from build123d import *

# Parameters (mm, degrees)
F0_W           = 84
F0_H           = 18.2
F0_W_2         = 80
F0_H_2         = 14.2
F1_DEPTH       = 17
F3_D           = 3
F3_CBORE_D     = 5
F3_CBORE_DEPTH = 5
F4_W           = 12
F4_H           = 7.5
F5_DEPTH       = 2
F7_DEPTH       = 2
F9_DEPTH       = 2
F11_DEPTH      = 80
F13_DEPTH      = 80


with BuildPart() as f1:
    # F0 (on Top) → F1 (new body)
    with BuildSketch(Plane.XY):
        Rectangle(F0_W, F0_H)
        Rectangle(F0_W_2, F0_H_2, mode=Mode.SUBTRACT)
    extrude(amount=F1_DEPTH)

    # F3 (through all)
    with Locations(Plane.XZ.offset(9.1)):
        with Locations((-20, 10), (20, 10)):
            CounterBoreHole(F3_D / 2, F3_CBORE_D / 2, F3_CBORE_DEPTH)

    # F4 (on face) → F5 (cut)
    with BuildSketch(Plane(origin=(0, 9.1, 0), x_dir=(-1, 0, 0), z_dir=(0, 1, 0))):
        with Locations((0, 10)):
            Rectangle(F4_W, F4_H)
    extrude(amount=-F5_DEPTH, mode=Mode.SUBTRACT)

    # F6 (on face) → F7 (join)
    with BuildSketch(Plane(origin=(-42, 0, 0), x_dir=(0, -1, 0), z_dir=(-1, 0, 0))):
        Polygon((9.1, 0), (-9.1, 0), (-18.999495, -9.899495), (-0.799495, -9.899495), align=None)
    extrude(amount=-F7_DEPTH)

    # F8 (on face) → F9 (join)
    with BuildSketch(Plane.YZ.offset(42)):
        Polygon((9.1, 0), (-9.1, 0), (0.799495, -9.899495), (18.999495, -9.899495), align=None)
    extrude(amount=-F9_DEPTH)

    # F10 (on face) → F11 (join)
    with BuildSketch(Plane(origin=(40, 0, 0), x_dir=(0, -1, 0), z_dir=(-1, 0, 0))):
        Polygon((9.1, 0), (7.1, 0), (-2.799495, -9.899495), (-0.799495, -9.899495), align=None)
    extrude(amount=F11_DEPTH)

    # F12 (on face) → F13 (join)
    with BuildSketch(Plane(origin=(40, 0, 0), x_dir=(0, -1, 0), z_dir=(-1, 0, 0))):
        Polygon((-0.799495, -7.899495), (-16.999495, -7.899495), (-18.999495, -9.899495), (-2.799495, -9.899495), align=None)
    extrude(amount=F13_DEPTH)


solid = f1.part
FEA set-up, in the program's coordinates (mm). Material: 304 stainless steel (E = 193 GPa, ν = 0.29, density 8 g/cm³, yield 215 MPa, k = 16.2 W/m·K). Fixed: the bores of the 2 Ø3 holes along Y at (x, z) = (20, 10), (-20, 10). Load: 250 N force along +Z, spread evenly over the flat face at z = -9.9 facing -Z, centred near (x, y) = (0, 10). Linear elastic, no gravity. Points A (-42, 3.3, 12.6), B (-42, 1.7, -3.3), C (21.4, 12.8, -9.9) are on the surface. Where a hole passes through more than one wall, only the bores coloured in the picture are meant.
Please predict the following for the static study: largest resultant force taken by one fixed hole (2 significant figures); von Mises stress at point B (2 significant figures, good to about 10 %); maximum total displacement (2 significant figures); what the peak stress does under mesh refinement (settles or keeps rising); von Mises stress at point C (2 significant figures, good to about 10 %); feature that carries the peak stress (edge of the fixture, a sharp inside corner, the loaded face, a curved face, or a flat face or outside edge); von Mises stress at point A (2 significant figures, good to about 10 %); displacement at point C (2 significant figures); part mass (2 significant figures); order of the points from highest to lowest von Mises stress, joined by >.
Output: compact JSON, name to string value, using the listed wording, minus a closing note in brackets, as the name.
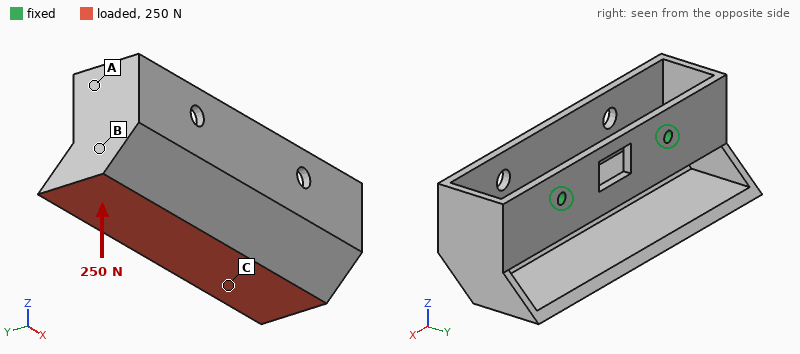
{"largest resultant force taken by one fixed hole": "150 N", "von Mises stress at point B": "20 MPa", "maximum total displacement": "0.12 mm", "what the peak stress does under mesh refinement": "keeps rising", "von Mises stress at point C": "32 MPa", "feature that carries the peak stress": "edge of the fixture", "von Mises stress at point A": "7.6 MPa", "displacement at point C": "0.065 mm", "part mass": "90 g", "order of the points from highest to lowest von Mises stress, joined by >": "C > B > A"}
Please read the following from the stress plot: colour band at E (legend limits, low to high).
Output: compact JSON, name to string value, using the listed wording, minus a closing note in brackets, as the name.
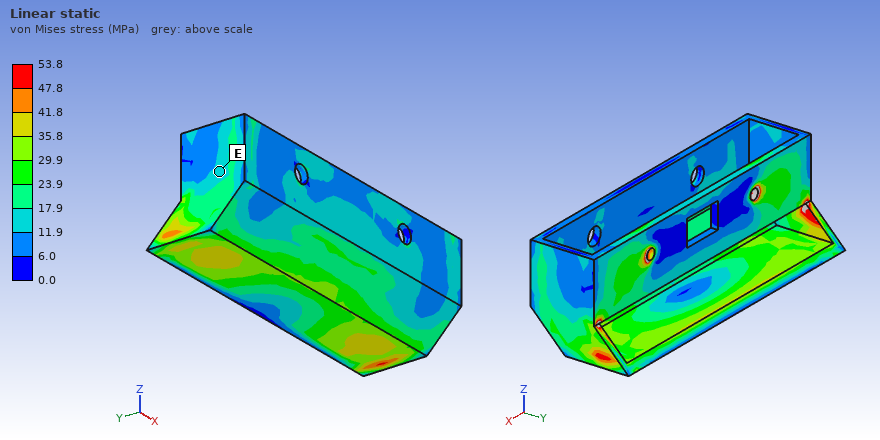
{"colour band at E": "11.9 to 17.9 MPa"}
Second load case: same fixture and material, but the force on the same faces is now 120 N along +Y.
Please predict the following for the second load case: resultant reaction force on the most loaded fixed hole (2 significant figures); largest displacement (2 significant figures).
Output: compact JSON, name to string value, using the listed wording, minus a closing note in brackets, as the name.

{"resultant reaction force on the most loaded fixed hole": "64 N", "largest displacement": "0.17 mm"}
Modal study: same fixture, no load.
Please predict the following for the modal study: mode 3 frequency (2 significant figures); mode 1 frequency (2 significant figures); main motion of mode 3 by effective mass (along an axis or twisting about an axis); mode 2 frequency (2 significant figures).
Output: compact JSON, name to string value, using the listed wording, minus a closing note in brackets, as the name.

{"mode 3 frequency": "1300 Hz", "mode 1 frequency": "640 Hz", "main motion of mode 3 by effective mass": "along Y", "mode 2 frequency": "940 Hz"}
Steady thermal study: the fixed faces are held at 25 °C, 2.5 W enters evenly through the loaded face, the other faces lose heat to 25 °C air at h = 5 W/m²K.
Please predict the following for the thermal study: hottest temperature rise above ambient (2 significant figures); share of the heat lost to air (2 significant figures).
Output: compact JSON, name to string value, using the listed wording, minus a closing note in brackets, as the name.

{"hottest temperature rise above ambient": "49 K", "share of the heat lost to air": "61 %"}
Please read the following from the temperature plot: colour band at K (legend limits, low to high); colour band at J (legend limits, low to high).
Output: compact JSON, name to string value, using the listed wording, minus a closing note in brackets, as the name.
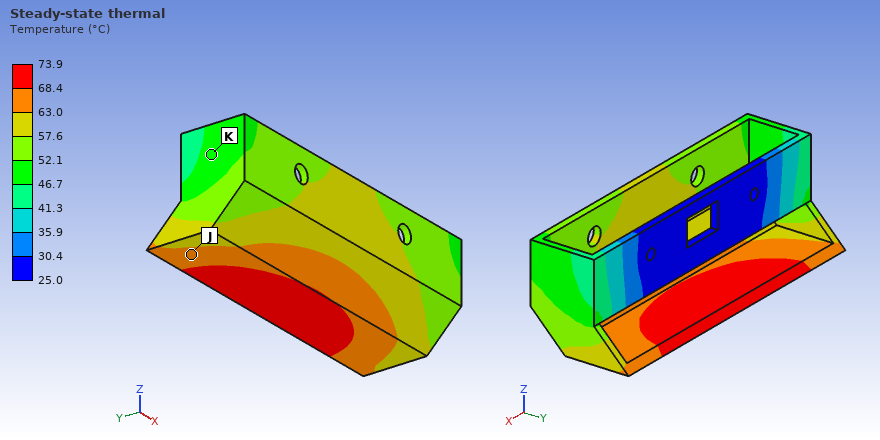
{"colour band at K": "46.7 to 52.1 °C", "colour band at J": "63.0 to 68.4 °C"}
